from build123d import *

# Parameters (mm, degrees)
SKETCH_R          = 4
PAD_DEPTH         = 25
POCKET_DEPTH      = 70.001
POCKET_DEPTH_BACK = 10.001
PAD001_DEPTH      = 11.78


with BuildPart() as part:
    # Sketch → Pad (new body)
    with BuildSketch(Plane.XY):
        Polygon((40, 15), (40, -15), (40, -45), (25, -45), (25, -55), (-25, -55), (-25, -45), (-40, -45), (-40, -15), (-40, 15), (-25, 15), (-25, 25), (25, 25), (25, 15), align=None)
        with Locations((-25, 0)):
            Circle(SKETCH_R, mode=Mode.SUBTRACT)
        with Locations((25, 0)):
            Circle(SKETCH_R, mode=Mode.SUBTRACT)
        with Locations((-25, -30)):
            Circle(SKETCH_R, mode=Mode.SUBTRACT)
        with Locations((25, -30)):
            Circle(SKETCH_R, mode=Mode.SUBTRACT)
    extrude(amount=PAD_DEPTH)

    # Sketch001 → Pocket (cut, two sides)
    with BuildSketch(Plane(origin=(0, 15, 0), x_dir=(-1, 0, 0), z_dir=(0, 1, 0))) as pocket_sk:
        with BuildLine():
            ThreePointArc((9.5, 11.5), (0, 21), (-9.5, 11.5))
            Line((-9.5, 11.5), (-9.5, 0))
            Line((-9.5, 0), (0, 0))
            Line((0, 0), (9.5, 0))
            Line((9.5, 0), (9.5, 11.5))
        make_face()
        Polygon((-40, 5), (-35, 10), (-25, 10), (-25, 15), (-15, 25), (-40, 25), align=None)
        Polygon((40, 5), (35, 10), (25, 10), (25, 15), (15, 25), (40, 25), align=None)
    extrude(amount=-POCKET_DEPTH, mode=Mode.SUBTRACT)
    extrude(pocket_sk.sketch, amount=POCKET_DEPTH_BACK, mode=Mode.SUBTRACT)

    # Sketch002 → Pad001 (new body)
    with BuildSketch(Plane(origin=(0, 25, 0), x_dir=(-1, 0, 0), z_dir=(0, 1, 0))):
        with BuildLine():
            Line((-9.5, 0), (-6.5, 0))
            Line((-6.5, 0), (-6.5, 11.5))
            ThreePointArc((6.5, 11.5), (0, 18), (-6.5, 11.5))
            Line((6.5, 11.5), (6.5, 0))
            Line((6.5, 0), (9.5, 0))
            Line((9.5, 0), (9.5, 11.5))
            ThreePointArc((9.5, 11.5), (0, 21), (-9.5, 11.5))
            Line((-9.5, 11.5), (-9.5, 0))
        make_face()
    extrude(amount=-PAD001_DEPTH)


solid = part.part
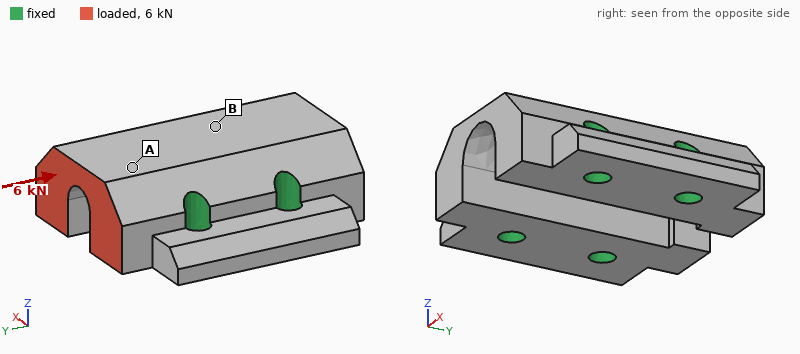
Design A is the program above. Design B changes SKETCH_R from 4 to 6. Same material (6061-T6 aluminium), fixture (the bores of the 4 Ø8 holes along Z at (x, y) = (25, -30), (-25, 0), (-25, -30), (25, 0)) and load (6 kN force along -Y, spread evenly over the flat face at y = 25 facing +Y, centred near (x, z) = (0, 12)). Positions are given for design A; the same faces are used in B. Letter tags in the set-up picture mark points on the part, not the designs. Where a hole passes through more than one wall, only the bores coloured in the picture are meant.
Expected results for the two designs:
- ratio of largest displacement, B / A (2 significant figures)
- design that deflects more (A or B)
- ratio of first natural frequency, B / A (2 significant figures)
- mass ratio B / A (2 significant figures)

0.85
A
1.2
0.95
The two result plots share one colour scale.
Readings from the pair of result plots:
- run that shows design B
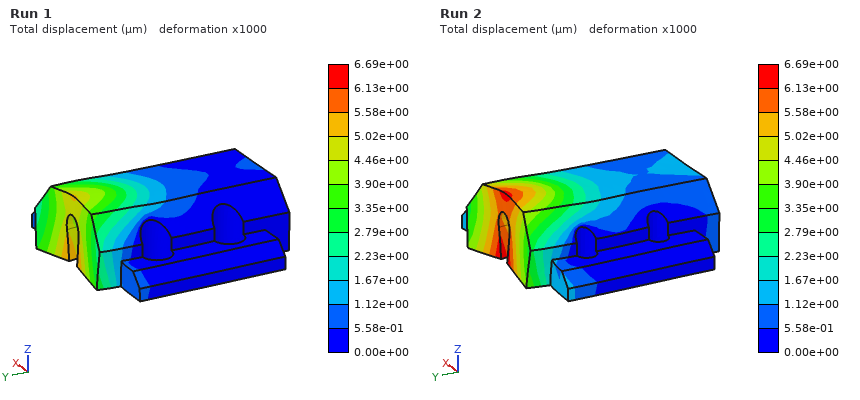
Run 1
